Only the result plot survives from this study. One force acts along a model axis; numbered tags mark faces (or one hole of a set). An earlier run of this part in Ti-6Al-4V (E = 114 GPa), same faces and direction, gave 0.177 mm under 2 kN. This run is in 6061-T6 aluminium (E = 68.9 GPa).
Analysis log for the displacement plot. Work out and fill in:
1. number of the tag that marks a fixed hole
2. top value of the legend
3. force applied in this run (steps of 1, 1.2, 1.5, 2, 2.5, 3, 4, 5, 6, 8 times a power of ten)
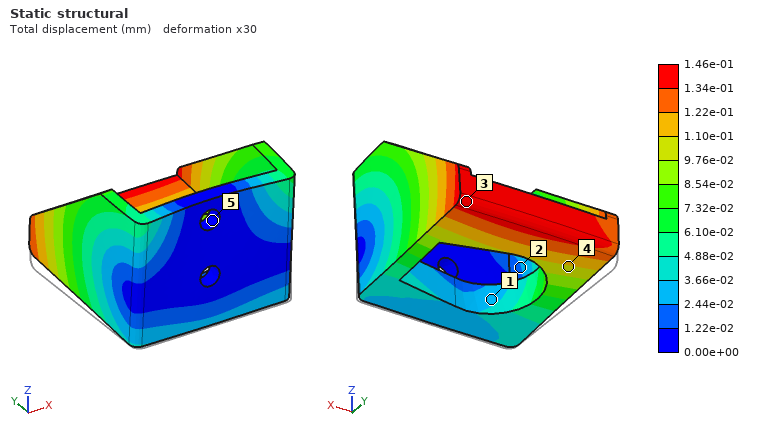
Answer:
5
1.46e-01 mm
1 kN
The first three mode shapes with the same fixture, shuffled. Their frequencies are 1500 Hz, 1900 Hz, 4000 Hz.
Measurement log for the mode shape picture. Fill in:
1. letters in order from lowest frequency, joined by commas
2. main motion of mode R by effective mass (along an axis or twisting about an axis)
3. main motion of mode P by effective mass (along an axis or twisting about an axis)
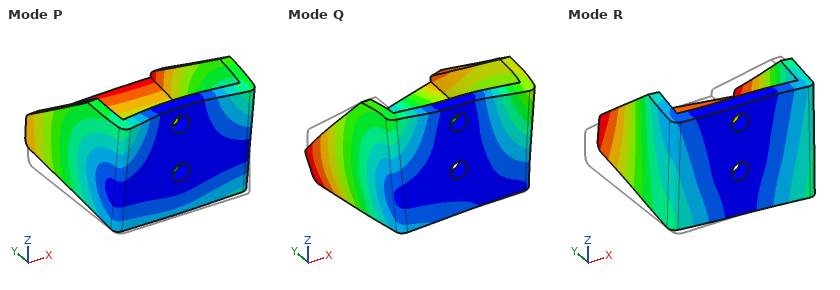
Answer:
R, P, Q
along X
along Z
